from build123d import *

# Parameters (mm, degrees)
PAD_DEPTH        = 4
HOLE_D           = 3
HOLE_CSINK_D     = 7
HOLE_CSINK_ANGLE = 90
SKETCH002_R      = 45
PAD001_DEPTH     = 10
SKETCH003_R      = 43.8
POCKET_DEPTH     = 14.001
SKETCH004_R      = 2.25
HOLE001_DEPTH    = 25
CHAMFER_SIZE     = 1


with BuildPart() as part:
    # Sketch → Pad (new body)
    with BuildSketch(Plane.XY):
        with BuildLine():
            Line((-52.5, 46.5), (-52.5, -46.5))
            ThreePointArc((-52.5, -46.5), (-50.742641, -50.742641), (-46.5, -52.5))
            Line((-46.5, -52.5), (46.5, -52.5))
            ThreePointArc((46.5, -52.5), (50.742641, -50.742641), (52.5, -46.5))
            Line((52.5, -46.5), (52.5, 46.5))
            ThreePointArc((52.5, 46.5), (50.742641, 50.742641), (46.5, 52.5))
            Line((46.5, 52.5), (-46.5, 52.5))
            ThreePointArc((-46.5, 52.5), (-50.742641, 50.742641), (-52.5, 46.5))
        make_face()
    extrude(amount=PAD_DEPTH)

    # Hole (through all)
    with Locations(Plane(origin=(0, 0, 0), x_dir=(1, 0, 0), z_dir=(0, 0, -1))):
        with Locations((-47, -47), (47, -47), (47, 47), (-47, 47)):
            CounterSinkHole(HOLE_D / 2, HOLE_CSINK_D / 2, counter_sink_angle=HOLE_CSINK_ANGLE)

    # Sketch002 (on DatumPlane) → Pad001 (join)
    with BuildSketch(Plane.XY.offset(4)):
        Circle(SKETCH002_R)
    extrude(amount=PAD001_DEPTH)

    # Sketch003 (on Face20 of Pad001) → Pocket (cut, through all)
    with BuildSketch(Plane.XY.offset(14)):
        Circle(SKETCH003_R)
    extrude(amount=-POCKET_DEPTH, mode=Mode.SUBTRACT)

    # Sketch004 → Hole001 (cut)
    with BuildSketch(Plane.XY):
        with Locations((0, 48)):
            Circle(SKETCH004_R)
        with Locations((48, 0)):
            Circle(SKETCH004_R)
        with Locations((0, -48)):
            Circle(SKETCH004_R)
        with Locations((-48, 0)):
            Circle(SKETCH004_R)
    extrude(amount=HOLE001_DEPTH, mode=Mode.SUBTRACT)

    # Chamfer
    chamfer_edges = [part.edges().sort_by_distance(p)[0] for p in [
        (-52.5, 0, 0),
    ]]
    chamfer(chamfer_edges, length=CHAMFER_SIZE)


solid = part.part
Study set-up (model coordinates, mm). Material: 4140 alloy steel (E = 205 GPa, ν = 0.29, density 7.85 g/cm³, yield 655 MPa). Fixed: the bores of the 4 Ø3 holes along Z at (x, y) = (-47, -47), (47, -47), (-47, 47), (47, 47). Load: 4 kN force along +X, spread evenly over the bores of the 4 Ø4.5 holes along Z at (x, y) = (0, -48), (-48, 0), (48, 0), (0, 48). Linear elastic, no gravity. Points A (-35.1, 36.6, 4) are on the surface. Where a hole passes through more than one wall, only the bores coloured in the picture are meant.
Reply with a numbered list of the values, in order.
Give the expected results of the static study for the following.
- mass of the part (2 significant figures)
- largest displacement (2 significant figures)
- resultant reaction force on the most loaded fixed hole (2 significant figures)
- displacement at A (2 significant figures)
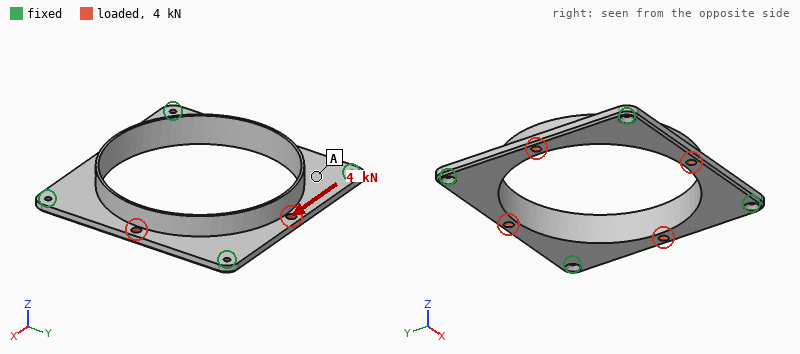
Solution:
1. 180 g
2. 37 µm
3. 1.0 kN
4. 9.8 µm
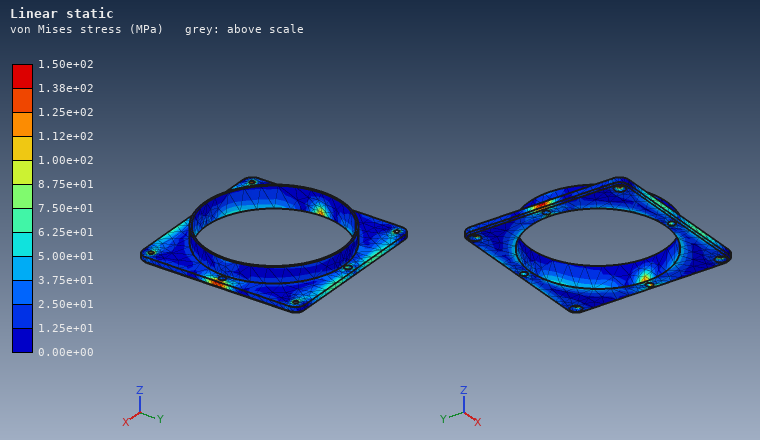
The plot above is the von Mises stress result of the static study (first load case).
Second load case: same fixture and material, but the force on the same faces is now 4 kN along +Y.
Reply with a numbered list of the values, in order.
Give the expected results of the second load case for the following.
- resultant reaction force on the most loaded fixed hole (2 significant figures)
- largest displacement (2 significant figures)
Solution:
1. 1.0 kN
2. 37 µm
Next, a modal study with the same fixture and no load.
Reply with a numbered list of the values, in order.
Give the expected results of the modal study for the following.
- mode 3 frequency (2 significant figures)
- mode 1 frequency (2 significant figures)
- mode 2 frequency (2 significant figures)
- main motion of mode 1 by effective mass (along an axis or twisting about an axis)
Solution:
1. 2500 Hz
2. 2300 Hz
3. 2500 Hz
4. along Z
